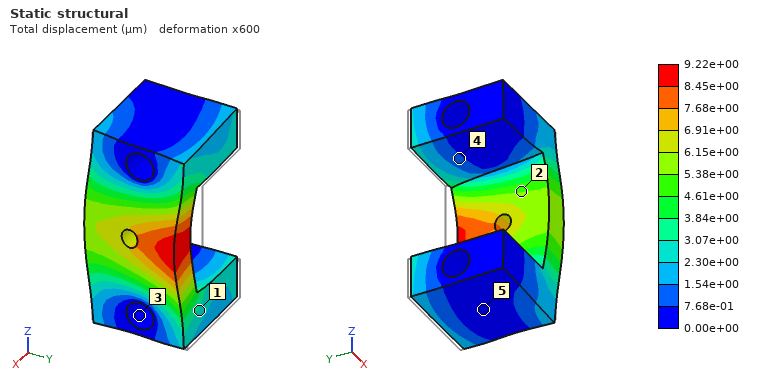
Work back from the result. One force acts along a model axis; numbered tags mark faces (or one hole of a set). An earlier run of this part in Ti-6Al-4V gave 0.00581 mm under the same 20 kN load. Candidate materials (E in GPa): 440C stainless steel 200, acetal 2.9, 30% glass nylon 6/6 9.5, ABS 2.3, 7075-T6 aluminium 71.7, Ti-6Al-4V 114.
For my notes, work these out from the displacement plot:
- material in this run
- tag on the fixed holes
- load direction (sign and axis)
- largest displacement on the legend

7075-T6 aluminium
3
-Y
9.22e+00 µm
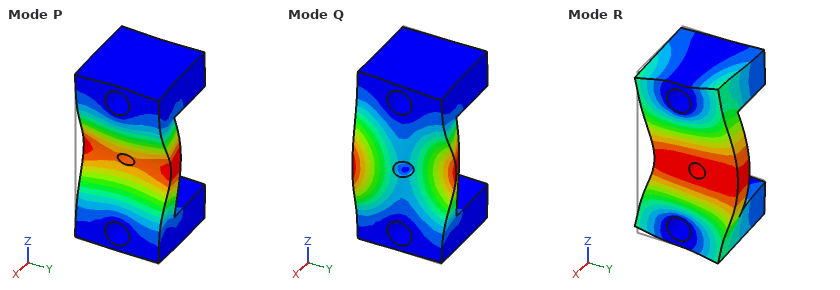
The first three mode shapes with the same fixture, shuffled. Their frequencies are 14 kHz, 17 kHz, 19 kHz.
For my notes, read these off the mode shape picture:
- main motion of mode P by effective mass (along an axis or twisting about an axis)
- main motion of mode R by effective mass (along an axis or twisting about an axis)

along X
along Y
